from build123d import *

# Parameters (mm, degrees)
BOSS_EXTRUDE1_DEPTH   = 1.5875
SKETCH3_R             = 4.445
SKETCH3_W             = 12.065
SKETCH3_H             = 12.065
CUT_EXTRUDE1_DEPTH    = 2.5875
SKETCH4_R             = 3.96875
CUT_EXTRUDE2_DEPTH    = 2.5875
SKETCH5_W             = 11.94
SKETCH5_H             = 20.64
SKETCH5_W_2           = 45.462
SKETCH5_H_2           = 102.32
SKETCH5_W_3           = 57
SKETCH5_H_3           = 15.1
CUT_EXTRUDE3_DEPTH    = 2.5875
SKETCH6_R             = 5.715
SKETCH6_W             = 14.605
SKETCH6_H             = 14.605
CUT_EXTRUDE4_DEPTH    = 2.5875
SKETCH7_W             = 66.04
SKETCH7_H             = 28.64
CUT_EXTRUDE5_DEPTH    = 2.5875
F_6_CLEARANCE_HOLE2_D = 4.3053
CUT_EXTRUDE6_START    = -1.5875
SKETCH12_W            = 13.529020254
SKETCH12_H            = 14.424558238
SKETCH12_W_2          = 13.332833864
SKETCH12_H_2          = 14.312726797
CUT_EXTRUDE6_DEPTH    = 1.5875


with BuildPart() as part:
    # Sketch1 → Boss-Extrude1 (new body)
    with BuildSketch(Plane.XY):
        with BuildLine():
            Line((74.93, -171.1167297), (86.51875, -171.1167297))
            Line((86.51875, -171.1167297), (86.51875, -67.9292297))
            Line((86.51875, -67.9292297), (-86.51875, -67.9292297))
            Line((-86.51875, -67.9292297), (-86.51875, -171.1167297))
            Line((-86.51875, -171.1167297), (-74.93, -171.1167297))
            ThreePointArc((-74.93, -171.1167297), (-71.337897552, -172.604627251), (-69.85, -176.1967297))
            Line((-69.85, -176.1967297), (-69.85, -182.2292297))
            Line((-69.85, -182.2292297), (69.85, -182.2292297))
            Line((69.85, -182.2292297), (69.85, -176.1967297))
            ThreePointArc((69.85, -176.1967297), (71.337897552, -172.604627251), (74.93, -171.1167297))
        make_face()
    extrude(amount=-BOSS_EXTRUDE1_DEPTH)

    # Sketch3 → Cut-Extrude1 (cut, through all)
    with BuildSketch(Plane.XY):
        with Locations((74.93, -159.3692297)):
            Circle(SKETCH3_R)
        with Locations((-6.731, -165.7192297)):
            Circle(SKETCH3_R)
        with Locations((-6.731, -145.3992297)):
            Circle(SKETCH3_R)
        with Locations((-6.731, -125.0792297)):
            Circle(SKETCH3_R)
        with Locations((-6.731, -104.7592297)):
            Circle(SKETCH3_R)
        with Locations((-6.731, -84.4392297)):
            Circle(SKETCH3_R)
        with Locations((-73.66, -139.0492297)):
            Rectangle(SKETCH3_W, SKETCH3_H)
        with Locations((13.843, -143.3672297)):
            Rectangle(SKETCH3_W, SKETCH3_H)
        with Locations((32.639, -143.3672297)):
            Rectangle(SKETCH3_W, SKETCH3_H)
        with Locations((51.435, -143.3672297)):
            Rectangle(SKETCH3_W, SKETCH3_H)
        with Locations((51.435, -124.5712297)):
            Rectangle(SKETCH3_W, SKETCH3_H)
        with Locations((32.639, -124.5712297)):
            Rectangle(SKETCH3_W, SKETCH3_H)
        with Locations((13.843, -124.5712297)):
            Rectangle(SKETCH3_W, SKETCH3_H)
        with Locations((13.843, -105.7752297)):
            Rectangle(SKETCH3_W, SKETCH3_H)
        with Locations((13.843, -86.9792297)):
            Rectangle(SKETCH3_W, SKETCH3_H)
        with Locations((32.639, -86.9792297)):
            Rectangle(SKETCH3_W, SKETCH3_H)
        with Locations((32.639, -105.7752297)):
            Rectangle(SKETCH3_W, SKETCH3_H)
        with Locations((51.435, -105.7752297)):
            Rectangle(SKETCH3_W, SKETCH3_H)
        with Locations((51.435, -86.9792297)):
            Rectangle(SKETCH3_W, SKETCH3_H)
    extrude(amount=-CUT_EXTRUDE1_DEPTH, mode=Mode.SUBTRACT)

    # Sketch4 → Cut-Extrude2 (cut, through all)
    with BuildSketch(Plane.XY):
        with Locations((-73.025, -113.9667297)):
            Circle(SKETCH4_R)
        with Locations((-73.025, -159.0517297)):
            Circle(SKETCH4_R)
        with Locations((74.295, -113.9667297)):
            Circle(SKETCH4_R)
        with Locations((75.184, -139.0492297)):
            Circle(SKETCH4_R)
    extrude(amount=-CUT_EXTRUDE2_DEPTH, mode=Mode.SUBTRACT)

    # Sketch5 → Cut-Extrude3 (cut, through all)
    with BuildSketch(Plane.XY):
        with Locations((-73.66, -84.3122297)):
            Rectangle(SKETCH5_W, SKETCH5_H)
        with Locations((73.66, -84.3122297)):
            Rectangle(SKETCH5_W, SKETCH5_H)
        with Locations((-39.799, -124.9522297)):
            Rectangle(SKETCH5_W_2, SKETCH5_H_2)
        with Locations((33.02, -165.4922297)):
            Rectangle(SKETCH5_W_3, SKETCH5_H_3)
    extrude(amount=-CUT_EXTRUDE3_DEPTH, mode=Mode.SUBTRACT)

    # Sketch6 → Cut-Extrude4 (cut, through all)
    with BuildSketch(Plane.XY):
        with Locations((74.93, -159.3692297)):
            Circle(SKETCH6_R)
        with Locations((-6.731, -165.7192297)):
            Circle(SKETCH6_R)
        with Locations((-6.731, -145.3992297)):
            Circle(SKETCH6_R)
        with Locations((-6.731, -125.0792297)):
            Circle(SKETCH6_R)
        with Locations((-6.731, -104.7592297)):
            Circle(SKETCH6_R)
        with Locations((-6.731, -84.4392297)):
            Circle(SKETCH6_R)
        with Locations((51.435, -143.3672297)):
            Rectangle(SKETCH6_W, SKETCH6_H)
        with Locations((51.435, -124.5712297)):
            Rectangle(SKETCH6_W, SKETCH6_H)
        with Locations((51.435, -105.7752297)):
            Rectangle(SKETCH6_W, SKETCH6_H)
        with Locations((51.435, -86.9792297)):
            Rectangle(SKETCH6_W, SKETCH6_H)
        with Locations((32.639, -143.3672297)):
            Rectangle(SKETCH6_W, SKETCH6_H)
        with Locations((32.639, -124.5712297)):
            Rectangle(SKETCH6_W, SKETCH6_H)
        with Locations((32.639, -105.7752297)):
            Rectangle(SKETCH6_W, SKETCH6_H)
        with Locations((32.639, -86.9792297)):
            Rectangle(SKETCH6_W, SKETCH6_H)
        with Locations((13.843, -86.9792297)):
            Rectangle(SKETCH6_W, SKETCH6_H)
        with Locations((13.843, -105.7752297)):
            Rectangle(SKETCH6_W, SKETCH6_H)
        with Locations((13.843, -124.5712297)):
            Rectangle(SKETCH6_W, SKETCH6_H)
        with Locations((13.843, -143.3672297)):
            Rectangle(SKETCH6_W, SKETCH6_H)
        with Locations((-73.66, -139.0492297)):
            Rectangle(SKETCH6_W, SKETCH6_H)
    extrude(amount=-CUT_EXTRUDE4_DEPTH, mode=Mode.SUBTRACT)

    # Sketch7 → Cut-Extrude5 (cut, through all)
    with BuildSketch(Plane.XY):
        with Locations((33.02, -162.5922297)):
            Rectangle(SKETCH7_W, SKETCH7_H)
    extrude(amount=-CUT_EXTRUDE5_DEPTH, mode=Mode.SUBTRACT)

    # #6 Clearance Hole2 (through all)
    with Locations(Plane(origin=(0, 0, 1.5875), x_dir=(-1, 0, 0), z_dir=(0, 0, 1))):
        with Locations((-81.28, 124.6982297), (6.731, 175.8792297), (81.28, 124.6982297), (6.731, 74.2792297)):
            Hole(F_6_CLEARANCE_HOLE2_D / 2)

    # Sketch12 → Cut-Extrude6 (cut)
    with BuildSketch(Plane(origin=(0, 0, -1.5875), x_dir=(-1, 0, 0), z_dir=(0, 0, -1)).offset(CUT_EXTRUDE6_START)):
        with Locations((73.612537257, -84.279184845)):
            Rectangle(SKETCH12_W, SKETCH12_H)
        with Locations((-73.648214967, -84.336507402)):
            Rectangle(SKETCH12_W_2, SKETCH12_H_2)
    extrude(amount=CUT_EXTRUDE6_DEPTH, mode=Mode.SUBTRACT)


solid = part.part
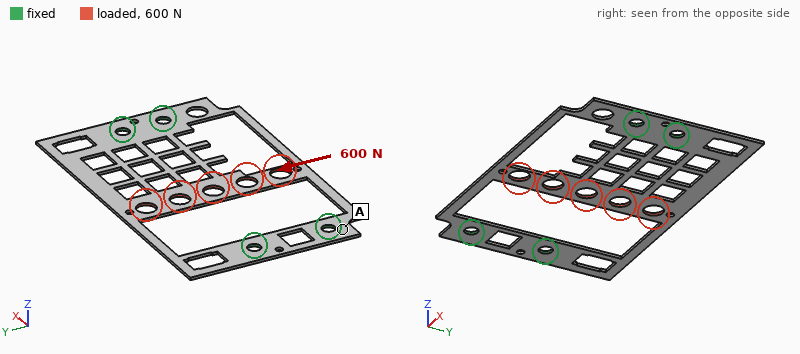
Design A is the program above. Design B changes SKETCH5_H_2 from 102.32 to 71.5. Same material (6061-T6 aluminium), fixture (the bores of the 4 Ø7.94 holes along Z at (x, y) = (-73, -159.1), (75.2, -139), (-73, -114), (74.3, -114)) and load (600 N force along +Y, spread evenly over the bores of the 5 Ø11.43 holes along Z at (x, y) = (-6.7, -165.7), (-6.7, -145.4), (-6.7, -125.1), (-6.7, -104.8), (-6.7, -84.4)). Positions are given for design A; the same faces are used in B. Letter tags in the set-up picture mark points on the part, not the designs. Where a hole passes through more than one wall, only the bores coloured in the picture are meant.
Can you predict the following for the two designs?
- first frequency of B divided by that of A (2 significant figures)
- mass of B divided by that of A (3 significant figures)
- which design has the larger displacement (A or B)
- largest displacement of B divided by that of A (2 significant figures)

1.1
1.16
A
0.35
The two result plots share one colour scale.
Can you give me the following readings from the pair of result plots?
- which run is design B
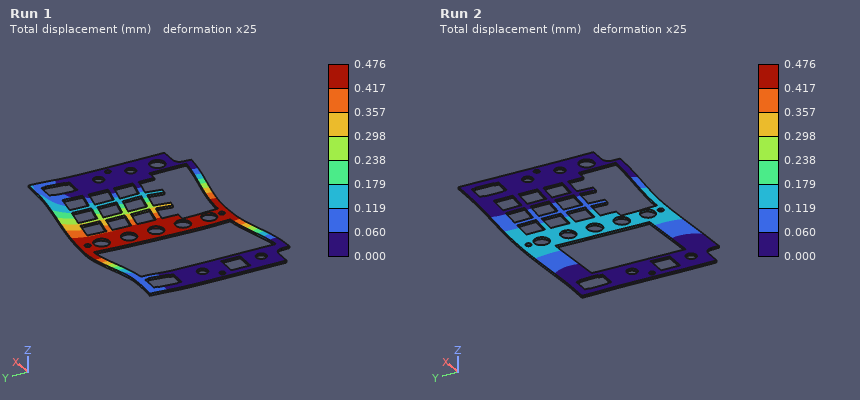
Run 2
